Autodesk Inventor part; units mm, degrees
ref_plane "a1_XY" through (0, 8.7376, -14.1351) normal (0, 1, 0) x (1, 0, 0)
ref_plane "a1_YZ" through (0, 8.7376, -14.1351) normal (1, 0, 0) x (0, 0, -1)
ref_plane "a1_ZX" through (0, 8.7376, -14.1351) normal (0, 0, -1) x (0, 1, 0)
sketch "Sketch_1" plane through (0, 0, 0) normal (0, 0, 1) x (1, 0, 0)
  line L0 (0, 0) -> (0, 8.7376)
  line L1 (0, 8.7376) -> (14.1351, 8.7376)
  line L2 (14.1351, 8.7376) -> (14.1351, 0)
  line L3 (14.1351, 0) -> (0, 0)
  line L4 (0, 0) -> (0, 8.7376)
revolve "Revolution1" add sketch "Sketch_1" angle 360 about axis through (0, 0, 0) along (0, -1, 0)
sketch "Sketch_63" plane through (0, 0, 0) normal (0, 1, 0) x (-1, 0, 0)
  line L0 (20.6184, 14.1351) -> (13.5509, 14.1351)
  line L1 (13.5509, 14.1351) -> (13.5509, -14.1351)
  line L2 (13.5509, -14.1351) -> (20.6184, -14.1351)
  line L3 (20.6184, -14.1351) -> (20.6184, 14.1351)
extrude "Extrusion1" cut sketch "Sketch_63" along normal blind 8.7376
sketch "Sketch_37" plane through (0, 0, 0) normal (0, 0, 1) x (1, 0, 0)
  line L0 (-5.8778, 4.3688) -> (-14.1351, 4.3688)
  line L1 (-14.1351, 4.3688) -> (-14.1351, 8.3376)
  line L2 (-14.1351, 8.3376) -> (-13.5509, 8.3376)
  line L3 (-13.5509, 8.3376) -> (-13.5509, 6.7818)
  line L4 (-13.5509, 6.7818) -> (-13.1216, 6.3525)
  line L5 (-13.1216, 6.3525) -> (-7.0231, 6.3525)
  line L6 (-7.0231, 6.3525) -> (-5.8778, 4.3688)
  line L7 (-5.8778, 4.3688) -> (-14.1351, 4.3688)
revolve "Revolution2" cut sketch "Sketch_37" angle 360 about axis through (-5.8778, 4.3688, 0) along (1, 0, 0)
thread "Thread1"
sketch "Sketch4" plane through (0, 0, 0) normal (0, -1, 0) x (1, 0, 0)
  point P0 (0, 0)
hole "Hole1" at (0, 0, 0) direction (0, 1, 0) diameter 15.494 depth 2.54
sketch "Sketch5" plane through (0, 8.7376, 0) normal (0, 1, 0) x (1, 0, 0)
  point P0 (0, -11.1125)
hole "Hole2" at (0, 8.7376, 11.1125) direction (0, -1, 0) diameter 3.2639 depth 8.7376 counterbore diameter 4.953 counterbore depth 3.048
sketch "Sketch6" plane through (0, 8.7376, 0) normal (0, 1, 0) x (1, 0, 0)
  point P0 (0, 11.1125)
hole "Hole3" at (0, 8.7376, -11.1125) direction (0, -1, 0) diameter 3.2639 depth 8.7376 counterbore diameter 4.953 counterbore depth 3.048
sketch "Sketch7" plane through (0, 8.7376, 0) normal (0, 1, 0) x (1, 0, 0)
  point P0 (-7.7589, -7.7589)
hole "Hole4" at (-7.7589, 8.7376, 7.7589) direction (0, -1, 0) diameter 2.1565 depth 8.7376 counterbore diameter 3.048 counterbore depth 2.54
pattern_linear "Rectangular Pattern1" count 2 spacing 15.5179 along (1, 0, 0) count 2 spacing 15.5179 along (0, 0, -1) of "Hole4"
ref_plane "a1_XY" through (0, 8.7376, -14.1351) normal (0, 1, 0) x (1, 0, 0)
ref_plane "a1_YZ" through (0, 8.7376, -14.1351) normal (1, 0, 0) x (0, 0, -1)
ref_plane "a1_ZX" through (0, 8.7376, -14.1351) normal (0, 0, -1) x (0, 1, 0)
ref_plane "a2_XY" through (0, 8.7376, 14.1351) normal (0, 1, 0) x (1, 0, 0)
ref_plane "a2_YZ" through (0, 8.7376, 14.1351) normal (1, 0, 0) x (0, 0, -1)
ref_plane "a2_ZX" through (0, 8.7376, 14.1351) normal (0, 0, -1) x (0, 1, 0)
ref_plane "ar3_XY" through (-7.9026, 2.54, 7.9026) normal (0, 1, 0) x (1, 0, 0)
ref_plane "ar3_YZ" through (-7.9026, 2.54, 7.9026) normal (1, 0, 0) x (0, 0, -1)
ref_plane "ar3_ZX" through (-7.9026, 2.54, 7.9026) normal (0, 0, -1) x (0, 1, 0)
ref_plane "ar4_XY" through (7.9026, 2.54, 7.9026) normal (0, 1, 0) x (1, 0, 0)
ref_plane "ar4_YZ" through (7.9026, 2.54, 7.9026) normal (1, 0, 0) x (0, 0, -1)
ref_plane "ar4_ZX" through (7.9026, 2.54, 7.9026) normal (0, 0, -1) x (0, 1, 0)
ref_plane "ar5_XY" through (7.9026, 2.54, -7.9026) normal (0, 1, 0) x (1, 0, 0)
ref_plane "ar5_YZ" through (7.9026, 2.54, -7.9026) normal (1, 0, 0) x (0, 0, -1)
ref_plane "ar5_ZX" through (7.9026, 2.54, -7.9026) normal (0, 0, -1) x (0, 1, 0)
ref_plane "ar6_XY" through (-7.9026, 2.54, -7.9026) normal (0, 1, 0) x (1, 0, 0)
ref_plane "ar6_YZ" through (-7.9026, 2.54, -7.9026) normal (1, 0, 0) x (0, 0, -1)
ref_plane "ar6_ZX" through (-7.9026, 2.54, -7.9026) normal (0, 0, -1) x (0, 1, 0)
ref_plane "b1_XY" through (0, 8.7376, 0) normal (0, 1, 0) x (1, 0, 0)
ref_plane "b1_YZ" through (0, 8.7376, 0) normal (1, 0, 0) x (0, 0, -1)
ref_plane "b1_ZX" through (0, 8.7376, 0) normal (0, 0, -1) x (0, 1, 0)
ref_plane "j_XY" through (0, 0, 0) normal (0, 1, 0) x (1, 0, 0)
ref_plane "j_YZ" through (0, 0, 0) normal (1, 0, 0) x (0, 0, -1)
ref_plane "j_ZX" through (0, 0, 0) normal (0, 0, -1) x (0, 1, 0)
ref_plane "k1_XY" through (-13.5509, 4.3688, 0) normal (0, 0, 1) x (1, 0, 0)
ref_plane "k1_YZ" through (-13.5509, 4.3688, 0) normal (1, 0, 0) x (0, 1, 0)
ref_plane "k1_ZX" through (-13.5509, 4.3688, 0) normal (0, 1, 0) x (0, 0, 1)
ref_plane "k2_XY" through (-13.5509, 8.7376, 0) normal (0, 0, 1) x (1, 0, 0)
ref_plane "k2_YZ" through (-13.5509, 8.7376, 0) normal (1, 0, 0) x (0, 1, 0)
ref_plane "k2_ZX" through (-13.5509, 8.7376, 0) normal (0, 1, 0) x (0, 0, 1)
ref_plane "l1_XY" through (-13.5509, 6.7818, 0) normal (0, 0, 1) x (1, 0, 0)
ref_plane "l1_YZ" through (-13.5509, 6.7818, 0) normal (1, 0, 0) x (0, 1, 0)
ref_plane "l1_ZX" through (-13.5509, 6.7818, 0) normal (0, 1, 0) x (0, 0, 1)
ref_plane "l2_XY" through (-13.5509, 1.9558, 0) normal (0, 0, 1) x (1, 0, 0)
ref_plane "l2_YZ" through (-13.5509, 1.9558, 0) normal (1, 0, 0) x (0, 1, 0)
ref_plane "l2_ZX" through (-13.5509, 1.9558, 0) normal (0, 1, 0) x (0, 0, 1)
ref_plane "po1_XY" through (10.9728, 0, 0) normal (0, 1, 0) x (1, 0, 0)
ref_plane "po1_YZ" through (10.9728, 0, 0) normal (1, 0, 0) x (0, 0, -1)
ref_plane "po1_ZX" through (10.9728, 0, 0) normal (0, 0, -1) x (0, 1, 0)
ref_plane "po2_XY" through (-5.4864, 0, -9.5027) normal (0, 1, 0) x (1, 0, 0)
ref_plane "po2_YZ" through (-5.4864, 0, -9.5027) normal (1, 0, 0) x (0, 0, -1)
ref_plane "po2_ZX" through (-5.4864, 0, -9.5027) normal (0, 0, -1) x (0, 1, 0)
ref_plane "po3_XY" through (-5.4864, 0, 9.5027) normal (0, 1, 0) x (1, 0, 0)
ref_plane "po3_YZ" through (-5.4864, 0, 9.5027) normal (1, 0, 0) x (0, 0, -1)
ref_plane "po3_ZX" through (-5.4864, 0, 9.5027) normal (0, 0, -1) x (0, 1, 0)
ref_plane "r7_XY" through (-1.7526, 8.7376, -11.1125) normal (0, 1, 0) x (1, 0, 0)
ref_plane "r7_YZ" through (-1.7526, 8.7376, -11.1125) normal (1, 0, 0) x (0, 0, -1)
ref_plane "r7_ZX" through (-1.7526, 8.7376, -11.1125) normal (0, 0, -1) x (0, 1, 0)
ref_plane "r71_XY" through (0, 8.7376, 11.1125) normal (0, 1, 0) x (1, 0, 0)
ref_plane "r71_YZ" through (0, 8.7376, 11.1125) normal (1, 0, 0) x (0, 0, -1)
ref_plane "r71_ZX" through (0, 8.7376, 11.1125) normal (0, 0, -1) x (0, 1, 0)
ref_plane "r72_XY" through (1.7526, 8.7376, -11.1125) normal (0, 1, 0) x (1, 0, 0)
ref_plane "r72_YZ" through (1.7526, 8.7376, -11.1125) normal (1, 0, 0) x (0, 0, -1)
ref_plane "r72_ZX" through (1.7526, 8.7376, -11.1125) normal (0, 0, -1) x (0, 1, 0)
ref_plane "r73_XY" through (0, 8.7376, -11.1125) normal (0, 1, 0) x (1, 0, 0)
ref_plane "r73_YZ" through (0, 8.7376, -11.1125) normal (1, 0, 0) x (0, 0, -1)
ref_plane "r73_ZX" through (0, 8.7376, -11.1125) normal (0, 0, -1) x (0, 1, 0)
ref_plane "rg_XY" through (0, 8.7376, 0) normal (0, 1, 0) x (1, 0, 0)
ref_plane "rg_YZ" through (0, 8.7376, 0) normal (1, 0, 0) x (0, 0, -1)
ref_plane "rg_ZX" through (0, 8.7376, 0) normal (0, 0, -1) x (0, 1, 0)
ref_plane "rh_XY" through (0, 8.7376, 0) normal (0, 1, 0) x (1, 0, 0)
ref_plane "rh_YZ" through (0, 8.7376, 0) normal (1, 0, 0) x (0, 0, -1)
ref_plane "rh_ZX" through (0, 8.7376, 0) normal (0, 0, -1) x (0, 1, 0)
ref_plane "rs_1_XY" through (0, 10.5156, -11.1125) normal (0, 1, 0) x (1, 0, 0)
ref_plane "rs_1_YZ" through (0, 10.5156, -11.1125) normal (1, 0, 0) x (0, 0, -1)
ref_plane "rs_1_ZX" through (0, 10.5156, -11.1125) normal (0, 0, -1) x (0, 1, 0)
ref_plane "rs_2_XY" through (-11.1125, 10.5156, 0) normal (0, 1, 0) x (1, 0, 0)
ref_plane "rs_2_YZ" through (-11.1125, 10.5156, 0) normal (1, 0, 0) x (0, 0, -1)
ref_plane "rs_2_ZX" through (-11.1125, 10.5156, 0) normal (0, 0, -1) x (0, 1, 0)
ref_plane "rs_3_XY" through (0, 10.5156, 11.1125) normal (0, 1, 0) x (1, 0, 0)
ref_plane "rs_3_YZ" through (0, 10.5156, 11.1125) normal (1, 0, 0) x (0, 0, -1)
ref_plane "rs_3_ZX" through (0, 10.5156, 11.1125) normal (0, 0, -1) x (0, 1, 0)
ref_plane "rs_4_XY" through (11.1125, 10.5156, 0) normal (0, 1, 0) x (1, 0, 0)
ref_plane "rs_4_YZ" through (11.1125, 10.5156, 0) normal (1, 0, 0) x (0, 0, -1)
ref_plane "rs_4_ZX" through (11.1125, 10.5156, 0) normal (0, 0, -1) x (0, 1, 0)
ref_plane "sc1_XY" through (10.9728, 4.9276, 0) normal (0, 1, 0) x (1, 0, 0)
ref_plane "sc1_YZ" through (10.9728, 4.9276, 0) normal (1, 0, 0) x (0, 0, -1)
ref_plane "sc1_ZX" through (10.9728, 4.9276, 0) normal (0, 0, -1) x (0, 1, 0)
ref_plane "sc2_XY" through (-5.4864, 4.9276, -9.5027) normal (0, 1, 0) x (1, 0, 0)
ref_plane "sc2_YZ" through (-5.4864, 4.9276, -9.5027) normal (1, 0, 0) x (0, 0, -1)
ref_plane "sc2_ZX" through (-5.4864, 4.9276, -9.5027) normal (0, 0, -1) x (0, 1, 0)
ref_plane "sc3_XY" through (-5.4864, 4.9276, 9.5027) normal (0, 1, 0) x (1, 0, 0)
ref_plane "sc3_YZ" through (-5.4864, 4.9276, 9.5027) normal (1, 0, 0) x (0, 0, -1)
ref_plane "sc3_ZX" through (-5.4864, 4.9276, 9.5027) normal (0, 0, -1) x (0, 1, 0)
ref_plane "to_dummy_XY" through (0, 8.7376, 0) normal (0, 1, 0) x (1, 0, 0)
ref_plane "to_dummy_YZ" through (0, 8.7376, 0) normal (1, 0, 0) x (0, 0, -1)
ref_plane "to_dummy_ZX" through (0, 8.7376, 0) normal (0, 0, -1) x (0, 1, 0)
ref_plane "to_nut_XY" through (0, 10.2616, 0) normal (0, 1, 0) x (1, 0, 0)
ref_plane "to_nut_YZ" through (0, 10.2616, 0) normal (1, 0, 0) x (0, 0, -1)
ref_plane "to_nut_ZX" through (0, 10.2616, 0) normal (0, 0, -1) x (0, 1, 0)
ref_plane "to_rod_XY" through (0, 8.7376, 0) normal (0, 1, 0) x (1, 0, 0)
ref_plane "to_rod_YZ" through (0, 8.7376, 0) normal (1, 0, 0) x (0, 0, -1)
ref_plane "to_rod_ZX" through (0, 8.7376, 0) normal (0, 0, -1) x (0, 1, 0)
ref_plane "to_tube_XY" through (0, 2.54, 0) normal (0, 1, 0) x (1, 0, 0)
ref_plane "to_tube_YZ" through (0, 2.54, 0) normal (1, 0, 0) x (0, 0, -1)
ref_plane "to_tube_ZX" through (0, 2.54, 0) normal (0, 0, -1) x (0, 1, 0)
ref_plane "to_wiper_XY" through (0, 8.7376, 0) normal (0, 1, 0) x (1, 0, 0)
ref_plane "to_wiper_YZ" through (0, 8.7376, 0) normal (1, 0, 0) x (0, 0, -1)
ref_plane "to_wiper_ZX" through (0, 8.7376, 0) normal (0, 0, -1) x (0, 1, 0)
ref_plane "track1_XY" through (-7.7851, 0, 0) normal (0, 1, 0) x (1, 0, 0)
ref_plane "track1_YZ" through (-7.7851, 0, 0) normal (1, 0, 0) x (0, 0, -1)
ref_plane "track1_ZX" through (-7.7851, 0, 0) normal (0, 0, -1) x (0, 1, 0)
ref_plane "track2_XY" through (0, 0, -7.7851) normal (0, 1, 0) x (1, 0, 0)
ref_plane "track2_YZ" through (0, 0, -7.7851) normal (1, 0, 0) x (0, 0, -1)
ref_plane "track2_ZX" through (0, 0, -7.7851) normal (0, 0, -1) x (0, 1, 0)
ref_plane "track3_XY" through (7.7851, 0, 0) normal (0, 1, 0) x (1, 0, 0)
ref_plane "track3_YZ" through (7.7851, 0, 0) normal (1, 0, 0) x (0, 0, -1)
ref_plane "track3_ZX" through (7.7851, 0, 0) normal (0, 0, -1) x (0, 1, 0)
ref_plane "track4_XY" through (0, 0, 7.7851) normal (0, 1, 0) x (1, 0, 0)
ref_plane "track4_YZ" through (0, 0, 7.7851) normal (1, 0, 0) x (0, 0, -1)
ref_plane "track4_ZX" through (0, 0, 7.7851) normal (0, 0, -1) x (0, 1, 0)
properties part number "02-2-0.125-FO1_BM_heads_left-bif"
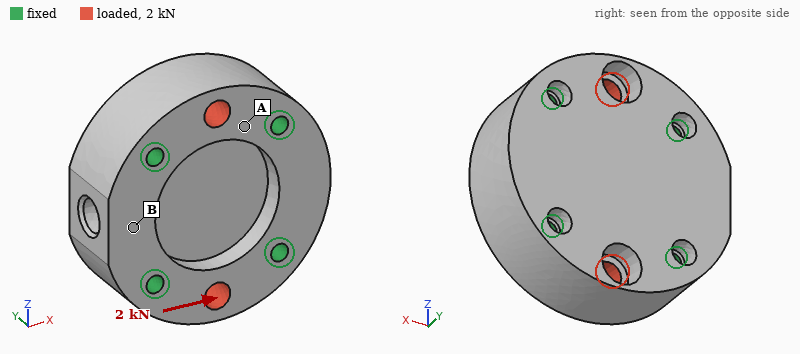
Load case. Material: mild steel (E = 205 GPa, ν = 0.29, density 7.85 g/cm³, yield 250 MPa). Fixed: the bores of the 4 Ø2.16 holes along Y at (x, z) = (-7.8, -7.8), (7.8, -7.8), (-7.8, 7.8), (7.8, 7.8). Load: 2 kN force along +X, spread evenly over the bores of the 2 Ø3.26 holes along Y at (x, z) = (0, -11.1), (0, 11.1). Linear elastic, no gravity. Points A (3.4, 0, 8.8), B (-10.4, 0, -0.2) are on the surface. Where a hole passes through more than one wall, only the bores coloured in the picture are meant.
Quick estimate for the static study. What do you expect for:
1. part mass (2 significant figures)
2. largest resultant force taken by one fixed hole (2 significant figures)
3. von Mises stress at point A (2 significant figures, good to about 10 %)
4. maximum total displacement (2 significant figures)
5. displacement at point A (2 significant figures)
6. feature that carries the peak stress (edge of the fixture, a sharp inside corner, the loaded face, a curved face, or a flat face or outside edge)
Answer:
35 g
520 N
13 MPa
0.97 µm
0.32 µm
edge of the fixture
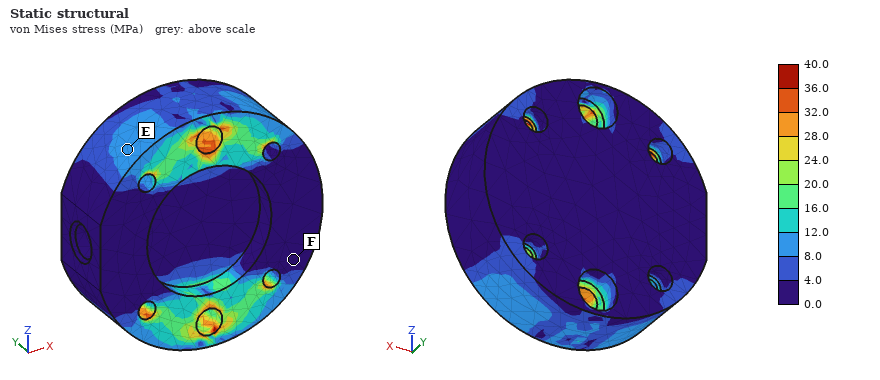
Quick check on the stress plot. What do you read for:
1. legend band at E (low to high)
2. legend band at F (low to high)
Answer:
8.0 to 12.0 MPa
0.0 to 4.0 MPa
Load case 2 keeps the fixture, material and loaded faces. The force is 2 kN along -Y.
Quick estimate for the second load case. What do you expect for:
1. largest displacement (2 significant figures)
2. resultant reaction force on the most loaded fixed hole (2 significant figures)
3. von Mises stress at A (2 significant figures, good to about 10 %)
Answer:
2.5 µm
530 N
22 MPa
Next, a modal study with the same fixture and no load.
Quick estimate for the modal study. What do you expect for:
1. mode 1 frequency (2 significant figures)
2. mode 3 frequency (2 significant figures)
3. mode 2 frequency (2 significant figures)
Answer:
60 kHz
65 kHz
61 kHz
